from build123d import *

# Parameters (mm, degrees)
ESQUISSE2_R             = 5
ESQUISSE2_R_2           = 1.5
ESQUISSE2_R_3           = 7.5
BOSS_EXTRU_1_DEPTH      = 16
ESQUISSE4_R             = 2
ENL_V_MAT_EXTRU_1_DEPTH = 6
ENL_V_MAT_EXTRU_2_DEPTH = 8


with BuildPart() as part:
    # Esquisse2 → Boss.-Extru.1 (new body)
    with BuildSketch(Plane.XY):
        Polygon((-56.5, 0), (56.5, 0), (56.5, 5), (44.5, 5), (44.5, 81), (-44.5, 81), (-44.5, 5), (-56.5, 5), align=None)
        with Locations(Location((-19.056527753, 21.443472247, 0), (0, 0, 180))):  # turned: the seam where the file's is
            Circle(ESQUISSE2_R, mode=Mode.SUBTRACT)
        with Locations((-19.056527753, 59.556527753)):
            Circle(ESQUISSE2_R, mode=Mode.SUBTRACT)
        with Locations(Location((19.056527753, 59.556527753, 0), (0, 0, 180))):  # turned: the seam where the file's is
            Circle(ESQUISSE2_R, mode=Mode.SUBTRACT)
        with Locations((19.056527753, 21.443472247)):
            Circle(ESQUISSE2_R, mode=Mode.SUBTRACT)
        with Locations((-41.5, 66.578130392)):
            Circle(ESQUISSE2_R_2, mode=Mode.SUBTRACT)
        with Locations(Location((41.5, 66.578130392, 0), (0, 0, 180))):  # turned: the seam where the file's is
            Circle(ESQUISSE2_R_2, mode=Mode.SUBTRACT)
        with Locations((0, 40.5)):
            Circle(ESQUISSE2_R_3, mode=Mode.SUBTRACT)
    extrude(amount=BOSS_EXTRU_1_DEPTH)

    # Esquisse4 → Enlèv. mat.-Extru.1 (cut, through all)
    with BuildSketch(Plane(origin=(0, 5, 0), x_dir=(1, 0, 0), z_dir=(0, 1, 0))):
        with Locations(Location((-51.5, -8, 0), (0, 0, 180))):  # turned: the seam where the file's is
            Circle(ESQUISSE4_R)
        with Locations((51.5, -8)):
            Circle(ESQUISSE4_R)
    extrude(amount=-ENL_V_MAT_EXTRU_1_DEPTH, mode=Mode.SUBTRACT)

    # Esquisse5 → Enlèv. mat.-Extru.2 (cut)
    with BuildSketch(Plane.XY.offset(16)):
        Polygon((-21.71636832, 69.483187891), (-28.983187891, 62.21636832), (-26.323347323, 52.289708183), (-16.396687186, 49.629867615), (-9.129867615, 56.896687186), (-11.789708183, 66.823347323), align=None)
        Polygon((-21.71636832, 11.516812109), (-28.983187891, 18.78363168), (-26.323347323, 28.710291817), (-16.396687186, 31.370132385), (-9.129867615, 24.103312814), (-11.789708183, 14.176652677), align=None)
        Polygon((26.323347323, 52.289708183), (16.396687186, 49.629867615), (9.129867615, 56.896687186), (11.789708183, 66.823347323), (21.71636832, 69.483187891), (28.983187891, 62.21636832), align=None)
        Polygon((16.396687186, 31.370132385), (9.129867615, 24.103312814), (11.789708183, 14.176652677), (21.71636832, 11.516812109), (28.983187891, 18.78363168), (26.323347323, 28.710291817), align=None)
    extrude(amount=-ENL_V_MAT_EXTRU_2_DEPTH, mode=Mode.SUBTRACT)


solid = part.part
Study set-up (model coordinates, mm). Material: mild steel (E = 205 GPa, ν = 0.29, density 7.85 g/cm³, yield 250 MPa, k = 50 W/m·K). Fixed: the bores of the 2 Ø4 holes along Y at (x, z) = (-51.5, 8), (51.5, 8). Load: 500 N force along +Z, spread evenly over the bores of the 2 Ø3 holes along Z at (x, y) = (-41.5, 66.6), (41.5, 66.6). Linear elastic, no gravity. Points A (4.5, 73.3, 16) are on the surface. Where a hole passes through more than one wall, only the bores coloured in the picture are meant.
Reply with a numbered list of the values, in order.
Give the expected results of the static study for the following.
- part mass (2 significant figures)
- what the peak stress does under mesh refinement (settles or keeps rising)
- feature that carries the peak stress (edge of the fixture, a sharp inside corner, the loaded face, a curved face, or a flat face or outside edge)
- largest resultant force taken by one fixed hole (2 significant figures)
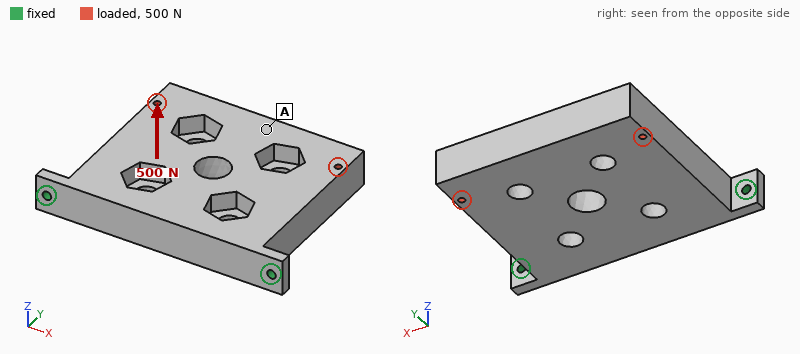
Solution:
1. 810 g
2. keeps rising
3. edge of the fixture
4. 250 N
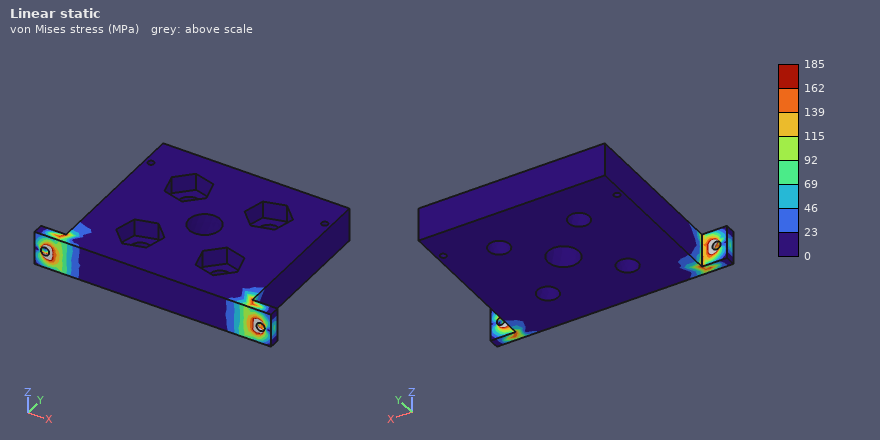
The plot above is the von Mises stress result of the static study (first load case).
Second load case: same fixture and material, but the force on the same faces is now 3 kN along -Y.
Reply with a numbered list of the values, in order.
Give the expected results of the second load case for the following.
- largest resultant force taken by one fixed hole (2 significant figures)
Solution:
1. 1.7 kN
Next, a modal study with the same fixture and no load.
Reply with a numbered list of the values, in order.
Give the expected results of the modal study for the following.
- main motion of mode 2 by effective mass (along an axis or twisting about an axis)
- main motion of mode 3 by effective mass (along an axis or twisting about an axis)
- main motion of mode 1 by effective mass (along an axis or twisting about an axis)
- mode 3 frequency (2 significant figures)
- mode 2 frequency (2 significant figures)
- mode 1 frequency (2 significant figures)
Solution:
1. twisting about Y
2. along X
3. along Z
4. 3200 Hz
5. 2900 Hz
6. 420 Hz
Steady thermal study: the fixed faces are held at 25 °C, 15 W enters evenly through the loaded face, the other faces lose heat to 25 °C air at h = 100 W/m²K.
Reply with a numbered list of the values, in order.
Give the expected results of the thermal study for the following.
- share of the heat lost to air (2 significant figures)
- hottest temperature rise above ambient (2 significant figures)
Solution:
1. 88 %
2. 15 K
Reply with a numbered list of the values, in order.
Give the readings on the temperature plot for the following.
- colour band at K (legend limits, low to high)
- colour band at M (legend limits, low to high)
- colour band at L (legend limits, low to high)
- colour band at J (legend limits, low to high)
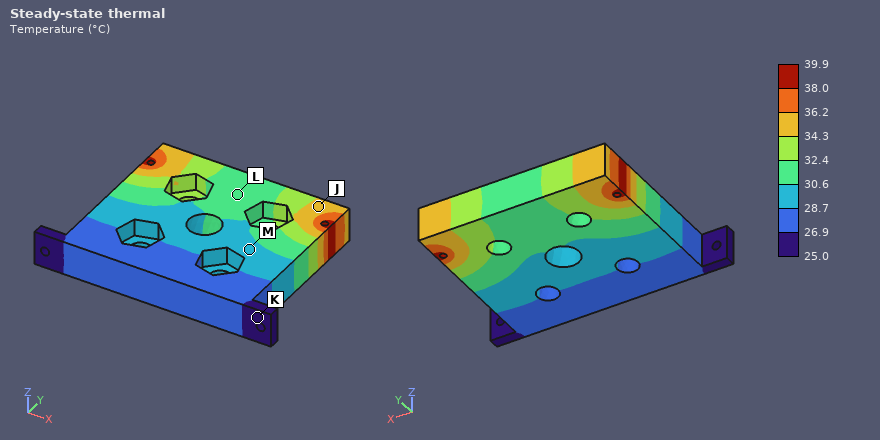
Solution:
1. 25.0 to 26.9 °C
2. 28.7 to 30.6 °C
3. 30.6 to 32.4 °C
4. 34.3 to 36.2 °C
